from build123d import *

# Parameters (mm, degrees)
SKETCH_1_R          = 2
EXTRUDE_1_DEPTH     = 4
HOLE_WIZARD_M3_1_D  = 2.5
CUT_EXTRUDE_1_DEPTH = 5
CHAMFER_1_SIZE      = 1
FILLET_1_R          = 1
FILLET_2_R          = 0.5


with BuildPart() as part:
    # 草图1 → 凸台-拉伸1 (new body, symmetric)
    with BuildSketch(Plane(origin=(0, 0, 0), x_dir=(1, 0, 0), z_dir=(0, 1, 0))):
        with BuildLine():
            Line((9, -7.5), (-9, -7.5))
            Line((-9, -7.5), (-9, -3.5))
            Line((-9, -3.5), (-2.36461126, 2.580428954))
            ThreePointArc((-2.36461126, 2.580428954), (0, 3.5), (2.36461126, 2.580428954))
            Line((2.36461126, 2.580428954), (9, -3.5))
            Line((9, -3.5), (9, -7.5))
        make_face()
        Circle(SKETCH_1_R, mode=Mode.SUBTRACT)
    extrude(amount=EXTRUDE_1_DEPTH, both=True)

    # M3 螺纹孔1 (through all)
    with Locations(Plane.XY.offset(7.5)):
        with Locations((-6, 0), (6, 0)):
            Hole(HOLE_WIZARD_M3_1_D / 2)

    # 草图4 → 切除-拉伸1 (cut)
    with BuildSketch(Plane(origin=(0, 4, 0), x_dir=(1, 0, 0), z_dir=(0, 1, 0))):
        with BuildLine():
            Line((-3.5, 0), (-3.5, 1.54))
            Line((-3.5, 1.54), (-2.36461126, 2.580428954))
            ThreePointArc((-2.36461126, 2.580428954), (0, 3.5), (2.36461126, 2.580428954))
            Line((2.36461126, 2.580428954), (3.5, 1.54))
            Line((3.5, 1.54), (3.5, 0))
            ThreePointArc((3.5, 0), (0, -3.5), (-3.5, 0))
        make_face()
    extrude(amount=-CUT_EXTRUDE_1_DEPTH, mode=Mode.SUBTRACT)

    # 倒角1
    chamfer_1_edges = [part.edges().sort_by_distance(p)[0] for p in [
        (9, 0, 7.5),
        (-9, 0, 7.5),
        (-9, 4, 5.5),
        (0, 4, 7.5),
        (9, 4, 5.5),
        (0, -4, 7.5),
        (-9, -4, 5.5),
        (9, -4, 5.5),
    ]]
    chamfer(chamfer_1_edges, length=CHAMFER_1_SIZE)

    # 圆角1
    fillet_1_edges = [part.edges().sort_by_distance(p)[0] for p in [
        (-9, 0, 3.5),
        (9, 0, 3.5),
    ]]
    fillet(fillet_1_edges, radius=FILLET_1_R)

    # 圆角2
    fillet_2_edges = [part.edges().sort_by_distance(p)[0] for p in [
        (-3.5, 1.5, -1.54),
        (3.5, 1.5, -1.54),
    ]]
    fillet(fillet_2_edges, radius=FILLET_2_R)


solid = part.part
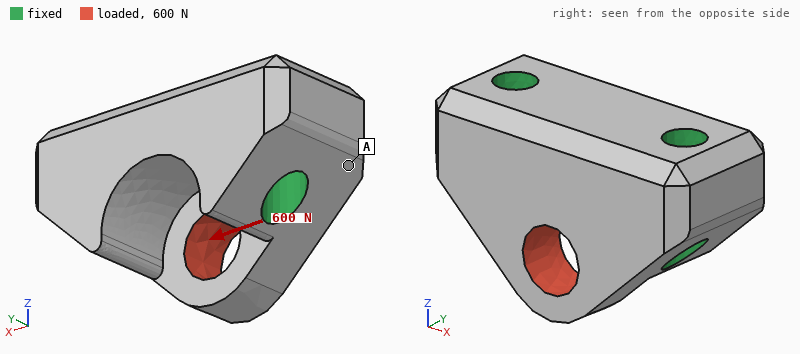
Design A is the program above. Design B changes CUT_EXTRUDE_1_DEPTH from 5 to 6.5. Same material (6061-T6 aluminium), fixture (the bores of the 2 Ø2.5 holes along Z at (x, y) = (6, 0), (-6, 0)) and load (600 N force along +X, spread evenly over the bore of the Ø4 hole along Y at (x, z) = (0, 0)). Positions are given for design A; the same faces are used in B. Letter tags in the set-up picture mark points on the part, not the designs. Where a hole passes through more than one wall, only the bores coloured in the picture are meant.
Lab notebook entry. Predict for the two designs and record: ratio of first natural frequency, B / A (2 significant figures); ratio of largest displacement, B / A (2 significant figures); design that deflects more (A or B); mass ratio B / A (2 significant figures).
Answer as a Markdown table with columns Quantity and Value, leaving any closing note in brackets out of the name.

| Quantity | Value |
|---|---|
| ratio of first natural frequency, B / A | 0.74 |
| ratio of largest displacement, B / A | 2.0 |
| design that deflects more | B |
| mass ratio B / A | 0.95 |
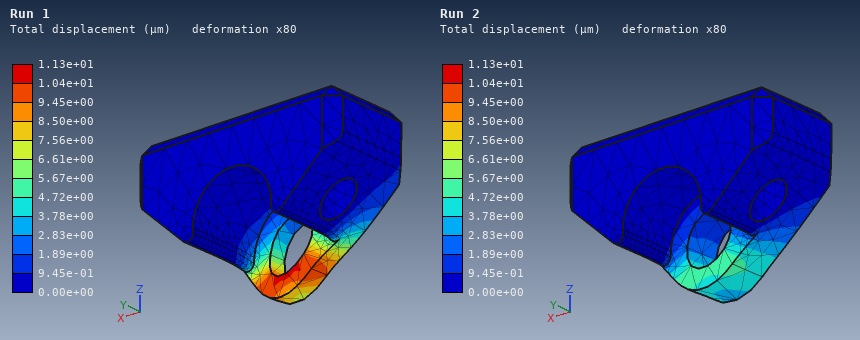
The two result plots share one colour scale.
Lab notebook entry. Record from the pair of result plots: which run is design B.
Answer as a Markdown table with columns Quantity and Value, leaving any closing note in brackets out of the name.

| Quantity | Value |
|---|---|
| which run is design B | Run 1 |
